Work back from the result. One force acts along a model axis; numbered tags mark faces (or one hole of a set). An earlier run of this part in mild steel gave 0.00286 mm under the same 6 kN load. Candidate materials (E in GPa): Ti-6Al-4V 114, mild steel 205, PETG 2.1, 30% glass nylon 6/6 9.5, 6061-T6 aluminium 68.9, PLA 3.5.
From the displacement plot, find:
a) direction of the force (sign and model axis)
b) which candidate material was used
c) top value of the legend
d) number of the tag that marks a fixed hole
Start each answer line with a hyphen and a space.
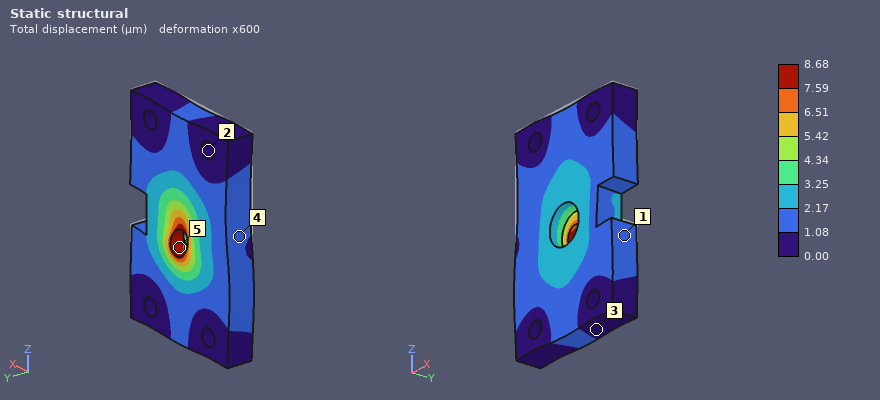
- -Z
- 6061-T6 aluminium
- 8.68 µm
- 2
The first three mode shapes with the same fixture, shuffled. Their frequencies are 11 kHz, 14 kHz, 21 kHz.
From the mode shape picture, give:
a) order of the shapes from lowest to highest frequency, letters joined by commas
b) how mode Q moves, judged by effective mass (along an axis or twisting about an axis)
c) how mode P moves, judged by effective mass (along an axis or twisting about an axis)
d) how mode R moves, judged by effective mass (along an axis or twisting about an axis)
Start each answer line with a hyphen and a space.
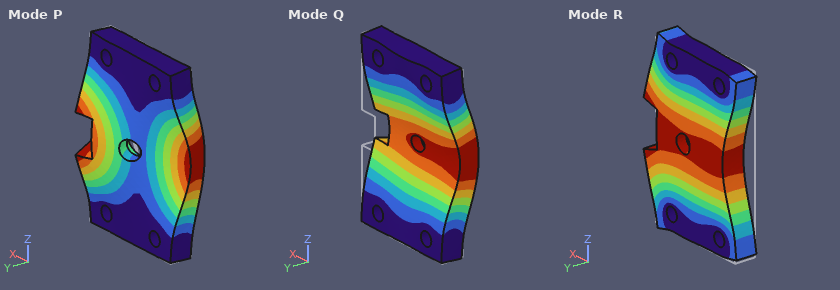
- Q, P, R
- along Y
- twisting about Z
- along X
